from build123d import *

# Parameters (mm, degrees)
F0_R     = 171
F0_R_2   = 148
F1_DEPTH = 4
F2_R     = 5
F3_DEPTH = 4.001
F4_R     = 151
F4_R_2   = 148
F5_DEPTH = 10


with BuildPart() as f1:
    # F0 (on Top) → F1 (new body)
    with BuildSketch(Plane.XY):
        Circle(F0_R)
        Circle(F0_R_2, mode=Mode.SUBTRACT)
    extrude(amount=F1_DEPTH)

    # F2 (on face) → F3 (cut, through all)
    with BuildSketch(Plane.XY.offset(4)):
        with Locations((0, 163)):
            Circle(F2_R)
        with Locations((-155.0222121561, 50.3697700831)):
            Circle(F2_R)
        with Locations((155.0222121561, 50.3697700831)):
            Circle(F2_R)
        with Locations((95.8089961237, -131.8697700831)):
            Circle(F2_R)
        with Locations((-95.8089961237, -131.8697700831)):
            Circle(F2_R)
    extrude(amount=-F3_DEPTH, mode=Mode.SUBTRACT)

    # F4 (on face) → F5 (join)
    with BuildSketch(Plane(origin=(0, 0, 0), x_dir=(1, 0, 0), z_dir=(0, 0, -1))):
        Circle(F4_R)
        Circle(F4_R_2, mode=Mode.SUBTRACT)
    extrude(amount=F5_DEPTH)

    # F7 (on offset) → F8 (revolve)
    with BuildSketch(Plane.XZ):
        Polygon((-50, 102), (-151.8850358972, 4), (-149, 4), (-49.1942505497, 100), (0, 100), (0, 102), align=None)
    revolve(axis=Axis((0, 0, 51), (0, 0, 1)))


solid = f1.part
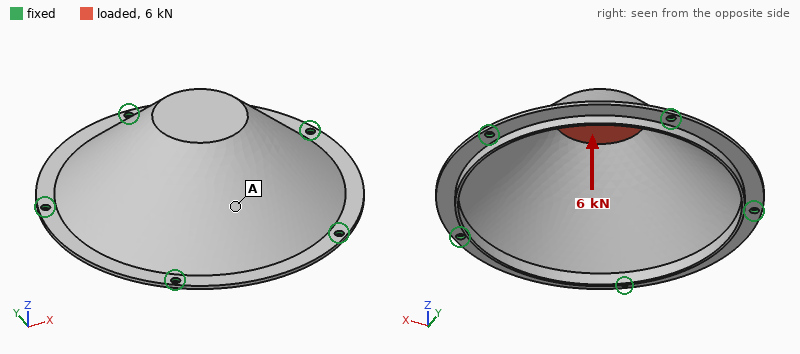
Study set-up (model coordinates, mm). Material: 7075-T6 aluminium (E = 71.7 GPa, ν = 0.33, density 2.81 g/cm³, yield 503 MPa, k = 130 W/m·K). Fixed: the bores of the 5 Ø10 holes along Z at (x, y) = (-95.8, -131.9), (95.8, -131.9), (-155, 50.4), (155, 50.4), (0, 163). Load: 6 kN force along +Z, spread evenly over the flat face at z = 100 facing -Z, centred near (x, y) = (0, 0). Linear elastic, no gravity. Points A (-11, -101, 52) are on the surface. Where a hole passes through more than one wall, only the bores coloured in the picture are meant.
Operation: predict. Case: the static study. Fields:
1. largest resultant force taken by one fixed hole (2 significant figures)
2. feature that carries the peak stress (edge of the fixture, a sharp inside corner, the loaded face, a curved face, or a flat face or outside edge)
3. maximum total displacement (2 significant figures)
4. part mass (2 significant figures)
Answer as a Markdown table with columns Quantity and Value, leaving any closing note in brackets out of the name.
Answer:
| Quantity | Value |
|---|---|
| largest resultant force taken by one fixed hole | 1.7 kN |
| feature that carries the peak stress | a flat face or outside edge |
| maximum total displacement | 1.9 mm |
| part mass | 870 g |
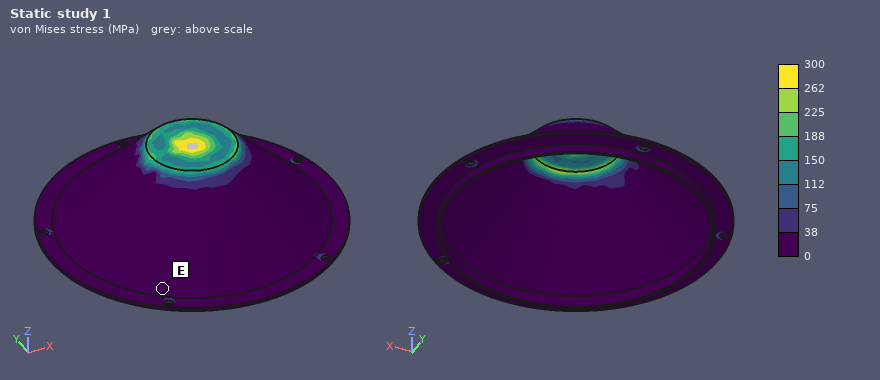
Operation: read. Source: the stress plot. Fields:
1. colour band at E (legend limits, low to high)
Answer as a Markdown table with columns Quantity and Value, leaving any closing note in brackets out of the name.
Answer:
| Quantity | Value |
|---|---|
| colour band at E | 0 to 38 MPa |
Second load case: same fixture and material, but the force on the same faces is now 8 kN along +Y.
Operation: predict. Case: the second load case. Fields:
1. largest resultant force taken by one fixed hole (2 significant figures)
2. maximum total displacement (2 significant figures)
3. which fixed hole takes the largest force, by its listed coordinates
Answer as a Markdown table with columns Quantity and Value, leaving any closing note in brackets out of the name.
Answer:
| Quantity | Value |
|---|---|
| largest resultant force taken by one fixed hole | 3.0 kN |
| maximum total displacement | 0.13 mm |
| which fixed hole takes the largest force, by its listed coordinates | (0, 163) |
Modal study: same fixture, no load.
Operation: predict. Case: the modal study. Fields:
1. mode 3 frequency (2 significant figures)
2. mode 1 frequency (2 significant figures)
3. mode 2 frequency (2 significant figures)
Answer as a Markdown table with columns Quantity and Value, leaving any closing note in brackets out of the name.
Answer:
| Quantity | Value |
|---|---|
| mode 3 frequency | 1700 Hz |
| mode 1 frequency | 1700 Hz |
| mode 2 frequency | 1700 Hz |
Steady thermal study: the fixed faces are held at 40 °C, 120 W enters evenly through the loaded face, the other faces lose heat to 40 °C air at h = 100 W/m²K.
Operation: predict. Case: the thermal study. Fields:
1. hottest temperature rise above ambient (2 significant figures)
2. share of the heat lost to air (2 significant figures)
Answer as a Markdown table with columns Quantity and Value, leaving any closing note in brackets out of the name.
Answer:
| Quantity | Value |
|---|---|
| hottest temperature rise above ambient | 56 K |
| share of the heat lost to air | 99 % |
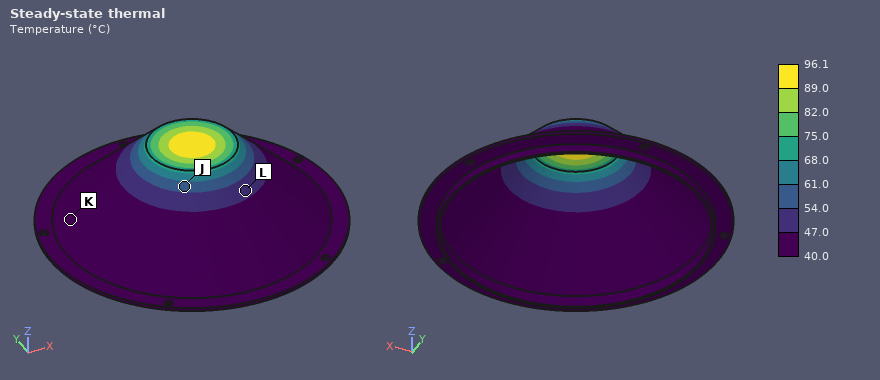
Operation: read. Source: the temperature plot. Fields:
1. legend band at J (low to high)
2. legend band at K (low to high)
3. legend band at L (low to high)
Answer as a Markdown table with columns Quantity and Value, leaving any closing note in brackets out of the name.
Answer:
| Quantity | Value |
|---|---|
| legend band at J | 54.0 to 61.0 °C |
| legend band at K | 40.0 to 47.0 °C |
| legend band at L | 47.0 to 54.0 °C |
